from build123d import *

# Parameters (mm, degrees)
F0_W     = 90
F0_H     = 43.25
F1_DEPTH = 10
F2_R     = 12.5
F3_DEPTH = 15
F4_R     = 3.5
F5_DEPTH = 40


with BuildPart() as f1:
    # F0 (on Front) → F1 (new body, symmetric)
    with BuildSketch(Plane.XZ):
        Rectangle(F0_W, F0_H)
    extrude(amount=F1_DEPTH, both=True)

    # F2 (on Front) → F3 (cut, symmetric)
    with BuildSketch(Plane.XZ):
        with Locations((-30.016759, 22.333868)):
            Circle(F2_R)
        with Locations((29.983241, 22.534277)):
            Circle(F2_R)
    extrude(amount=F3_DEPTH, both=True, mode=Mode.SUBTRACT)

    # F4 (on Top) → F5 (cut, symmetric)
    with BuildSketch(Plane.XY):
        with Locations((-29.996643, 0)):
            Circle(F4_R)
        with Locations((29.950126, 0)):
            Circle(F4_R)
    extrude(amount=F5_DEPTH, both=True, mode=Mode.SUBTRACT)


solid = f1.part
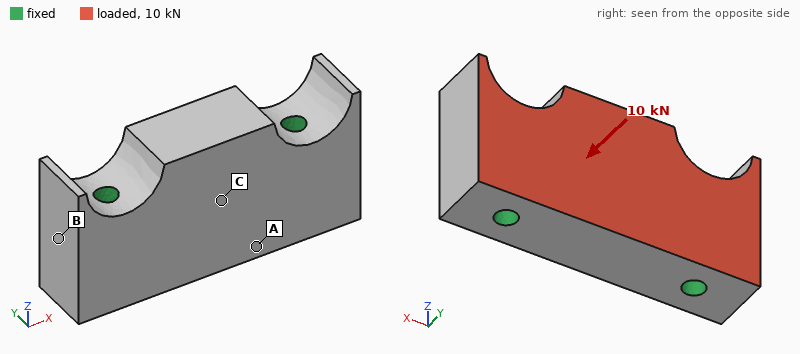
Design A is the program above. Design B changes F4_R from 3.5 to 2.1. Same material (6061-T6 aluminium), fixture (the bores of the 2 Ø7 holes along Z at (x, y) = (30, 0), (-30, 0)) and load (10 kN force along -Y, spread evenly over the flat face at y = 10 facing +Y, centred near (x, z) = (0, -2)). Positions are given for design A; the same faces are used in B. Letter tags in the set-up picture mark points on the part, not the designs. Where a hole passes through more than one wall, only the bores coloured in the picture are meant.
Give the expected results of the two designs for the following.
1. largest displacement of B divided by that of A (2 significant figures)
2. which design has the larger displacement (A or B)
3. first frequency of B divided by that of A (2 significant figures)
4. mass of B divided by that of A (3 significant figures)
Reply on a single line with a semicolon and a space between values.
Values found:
1.3; B; 0.84; 1.02
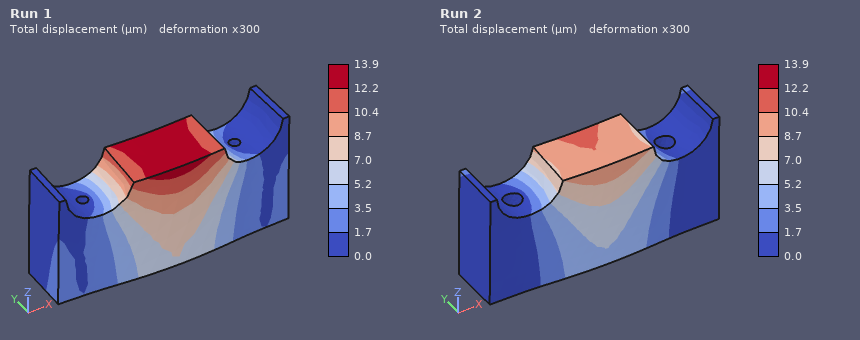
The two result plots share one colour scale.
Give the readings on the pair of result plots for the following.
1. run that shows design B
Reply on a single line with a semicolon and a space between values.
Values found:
Run 1
